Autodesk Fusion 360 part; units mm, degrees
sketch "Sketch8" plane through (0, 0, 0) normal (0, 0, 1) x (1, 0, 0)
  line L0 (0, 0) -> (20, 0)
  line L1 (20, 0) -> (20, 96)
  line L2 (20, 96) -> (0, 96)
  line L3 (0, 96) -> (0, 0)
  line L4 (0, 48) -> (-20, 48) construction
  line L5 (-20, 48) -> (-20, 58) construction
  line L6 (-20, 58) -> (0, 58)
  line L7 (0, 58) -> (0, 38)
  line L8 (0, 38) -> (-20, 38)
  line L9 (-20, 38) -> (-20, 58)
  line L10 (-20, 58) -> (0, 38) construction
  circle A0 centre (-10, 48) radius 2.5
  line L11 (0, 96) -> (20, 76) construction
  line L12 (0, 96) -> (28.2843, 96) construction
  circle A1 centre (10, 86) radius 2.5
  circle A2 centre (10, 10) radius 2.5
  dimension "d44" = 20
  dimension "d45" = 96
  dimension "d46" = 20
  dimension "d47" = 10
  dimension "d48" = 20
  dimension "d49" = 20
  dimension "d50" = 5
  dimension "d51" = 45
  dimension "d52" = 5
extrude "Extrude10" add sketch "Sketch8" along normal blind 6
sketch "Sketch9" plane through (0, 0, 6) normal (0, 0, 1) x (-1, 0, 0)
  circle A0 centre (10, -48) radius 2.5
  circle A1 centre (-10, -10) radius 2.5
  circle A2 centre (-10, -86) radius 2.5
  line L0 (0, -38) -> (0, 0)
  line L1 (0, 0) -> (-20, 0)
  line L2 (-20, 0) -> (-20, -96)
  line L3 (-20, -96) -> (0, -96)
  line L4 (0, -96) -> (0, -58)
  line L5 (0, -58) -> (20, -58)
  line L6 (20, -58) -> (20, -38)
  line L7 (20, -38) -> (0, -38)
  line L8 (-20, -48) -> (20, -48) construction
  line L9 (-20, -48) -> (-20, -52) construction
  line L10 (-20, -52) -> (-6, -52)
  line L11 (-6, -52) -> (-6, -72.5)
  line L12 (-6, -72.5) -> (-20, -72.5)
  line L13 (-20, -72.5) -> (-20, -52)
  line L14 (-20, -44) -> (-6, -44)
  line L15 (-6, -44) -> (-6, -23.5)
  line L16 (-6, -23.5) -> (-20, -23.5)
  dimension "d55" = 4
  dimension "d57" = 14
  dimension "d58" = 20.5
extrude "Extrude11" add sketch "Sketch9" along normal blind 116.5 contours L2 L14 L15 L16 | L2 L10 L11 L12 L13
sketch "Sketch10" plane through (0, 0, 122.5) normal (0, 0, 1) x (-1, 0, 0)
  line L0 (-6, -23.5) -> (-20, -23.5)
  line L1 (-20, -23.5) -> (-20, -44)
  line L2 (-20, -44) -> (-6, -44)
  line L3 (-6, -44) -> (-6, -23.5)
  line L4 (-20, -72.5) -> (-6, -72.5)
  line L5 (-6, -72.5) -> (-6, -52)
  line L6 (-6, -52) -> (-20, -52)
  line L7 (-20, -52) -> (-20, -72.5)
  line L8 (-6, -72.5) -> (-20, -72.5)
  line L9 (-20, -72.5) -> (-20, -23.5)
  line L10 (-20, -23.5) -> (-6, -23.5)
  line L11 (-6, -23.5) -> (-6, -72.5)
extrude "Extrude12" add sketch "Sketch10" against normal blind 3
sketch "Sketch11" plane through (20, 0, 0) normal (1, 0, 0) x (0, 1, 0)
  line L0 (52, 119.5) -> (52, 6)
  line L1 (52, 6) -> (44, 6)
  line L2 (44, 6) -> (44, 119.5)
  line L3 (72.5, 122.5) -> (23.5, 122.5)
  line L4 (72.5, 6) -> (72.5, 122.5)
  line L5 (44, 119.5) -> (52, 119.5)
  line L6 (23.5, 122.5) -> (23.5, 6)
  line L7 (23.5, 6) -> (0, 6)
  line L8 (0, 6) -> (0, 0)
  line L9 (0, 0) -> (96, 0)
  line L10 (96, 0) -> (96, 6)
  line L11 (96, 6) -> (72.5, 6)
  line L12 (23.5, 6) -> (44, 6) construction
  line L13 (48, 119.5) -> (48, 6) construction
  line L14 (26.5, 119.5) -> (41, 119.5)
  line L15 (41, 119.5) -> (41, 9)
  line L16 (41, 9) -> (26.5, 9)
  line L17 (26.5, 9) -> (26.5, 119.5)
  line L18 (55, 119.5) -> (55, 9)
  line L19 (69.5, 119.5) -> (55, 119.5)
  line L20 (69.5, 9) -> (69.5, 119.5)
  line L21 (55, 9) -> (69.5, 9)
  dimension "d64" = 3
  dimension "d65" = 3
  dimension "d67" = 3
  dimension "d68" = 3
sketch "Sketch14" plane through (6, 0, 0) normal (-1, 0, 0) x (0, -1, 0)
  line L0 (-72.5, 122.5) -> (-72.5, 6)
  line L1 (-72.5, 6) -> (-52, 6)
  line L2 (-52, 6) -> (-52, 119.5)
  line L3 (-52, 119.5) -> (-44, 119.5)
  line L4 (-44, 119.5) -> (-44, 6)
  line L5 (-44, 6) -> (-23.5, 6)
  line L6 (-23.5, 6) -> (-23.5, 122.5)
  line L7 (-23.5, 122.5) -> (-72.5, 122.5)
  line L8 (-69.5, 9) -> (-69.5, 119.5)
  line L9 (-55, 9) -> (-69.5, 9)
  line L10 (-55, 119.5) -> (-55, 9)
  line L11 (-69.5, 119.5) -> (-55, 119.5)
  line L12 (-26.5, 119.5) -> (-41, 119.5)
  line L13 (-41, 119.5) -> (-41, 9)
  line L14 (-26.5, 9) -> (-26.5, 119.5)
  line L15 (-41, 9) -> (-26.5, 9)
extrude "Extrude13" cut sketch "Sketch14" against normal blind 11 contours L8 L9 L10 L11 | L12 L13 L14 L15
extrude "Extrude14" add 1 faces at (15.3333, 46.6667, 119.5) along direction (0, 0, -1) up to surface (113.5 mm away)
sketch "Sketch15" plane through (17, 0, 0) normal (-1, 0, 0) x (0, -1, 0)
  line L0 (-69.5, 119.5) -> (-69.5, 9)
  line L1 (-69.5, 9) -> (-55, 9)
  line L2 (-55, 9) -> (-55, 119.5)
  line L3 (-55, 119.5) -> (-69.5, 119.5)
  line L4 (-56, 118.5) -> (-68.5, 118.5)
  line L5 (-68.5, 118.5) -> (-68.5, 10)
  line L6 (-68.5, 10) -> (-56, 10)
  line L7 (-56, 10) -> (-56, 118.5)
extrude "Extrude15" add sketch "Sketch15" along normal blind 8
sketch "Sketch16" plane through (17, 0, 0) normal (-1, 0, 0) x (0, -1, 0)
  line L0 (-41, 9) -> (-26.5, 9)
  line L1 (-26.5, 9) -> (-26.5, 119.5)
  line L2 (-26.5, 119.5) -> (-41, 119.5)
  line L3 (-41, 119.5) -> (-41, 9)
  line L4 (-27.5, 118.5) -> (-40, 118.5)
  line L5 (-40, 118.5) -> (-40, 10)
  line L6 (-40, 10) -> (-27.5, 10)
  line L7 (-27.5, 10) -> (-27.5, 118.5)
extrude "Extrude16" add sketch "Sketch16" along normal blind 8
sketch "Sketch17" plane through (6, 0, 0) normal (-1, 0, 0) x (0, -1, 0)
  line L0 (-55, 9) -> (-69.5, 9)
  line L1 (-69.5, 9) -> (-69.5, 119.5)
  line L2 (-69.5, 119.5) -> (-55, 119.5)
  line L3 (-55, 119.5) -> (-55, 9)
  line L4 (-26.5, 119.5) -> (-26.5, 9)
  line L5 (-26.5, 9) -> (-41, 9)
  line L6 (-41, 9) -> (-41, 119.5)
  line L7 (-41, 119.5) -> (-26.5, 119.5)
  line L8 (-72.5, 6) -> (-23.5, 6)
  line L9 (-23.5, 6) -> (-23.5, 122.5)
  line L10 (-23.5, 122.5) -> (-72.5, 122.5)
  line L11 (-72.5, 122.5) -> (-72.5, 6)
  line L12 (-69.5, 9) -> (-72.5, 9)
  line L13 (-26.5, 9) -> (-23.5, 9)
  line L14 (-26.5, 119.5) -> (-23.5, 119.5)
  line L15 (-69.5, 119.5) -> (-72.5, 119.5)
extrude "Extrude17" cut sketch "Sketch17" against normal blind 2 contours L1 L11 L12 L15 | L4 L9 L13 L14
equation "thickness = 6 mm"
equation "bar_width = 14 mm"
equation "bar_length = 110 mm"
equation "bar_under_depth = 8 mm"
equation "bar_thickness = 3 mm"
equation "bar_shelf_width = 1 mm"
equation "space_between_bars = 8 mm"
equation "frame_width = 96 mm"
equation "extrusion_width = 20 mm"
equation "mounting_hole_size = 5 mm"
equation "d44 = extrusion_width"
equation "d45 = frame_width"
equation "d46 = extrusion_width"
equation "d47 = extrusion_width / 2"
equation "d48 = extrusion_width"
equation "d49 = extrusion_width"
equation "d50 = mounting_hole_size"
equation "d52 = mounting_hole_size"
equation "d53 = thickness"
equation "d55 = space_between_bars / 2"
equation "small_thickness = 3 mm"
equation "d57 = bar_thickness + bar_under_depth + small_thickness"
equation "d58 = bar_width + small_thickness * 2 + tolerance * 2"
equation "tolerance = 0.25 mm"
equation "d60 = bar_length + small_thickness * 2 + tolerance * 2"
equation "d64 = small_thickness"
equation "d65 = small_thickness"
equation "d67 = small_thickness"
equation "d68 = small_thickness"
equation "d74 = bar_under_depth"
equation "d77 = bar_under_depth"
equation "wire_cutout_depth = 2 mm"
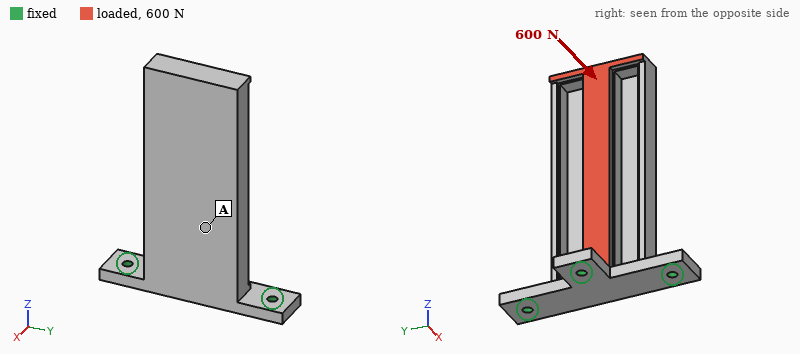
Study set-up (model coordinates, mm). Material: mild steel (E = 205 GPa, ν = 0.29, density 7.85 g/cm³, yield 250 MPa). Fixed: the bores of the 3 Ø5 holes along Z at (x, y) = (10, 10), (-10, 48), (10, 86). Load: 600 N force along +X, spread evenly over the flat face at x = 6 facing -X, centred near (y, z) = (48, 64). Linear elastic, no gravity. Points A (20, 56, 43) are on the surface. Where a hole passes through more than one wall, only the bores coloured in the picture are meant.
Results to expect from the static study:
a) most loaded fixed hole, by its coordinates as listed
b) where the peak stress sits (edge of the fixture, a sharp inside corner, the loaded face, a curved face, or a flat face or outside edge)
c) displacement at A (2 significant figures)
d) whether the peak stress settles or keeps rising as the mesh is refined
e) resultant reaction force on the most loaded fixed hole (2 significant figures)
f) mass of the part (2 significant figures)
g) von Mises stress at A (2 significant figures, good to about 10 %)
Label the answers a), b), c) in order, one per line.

a) (-10, 48)
b) edge of the fixture
c) 0.071 mm
d) keeps rising
e) 1.4 kN
f) 480 g
g) 15 MPa
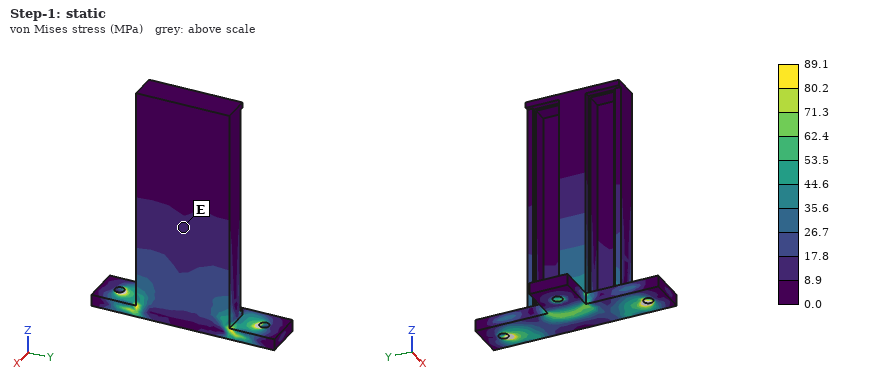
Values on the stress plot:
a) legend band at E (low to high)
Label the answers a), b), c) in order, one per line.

a) 8.9 to 17.8 MPa
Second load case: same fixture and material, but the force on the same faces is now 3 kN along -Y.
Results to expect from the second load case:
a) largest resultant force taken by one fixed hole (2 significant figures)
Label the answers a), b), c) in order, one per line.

a) 3.2 kN
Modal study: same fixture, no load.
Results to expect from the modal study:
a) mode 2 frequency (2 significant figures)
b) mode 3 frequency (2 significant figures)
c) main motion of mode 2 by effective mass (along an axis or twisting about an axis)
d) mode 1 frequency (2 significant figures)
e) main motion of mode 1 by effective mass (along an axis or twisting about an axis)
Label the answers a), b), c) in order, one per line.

a) 1300 Hz
b) 2400 Hz
c) along Y
d) 490 Hz
e) along X
